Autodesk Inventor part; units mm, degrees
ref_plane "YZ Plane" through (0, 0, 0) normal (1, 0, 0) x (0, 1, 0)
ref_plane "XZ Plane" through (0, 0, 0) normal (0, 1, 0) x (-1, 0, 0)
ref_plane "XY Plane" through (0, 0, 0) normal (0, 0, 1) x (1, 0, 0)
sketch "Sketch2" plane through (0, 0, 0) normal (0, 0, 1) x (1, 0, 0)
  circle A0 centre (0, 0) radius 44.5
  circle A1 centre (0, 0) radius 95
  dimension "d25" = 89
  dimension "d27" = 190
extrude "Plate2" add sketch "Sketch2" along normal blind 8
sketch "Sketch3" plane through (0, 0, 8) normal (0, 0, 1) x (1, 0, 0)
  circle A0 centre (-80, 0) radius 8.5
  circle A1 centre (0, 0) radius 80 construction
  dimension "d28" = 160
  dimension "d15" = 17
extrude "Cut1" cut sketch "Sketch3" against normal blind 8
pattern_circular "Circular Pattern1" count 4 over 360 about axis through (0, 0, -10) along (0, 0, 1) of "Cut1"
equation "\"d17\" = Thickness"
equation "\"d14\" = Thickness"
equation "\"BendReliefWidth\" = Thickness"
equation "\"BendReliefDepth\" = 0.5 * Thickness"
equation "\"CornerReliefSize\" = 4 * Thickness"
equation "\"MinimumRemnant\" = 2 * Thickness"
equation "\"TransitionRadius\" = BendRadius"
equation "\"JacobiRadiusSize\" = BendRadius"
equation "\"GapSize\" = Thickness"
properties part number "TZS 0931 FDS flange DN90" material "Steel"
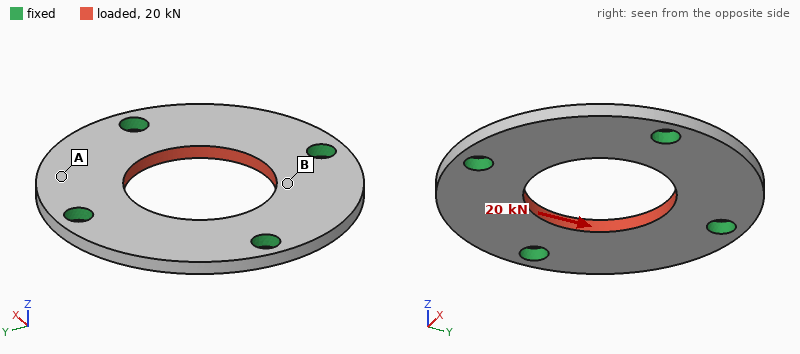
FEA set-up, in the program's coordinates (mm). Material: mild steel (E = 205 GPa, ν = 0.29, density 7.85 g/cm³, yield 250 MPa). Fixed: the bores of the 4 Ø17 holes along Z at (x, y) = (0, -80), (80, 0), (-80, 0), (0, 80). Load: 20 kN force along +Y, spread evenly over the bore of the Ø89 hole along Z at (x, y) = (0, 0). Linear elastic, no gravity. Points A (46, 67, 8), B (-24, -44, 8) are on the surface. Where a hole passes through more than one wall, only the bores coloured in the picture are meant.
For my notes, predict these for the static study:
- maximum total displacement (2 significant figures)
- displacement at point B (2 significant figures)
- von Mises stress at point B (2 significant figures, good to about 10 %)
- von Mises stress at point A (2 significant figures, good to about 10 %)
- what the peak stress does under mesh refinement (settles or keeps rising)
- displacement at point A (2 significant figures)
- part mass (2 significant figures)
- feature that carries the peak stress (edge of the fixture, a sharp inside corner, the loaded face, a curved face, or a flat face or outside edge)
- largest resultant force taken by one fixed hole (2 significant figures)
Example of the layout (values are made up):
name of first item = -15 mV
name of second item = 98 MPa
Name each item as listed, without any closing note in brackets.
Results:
maximum total displacement = 4.4 µm
displacement at point B = 3.3 µm
von Mises stress at point B = 13 MPa
von Mises stress at point A = 5.3 MPa
what the peak stress does under mesh refinement = keeps rising
displacement at point A = 3.0 µm
part mass = 1.3 kg
feature that carries the peak stress = edge of the fixture
largest resultant force taken by one fixed hole = 5.2 kN
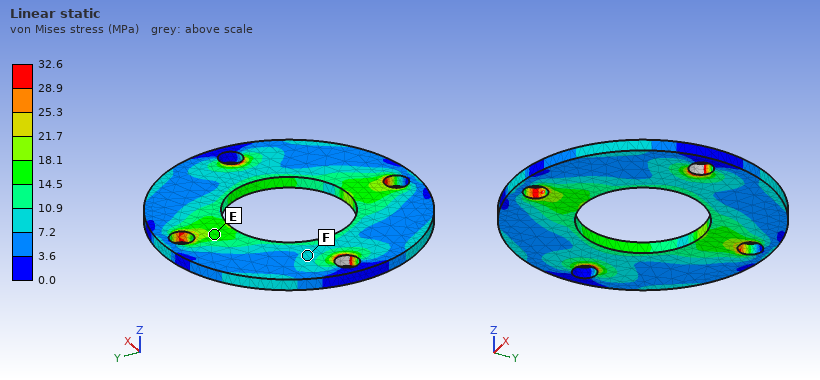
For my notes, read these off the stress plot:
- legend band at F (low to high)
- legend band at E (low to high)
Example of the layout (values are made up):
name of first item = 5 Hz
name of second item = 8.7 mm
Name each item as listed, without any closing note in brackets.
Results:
legend band at F = 7.2 to 10.9 MPa
legend band at E = 14.5 to 18.1 MPa
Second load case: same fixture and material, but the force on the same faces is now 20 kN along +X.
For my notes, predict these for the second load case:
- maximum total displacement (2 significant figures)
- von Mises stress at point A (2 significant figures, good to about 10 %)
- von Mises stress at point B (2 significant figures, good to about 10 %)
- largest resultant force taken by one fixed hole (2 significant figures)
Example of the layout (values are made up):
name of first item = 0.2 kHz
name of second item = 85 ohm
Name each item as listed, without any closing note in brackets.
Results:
maximum total displacement = 4.4 µm
von Mises stress at point A = 6.5 MPa
von Mises stress at point B = 9.2 MPa
largest resultant force taken by one fixed hole = 5.2 kN
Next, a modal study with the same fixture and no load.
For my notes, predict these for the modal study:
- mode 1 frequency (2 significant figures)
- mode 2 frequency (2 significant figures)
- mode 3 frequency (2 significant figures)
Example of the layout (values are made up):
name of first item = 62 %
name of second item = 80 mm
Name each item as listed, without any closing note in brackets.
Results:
mode 1 frequency = 3000 Hz
mode 2 frequency = 3100 Hz
mode 3 frequency = 3100 Hz
